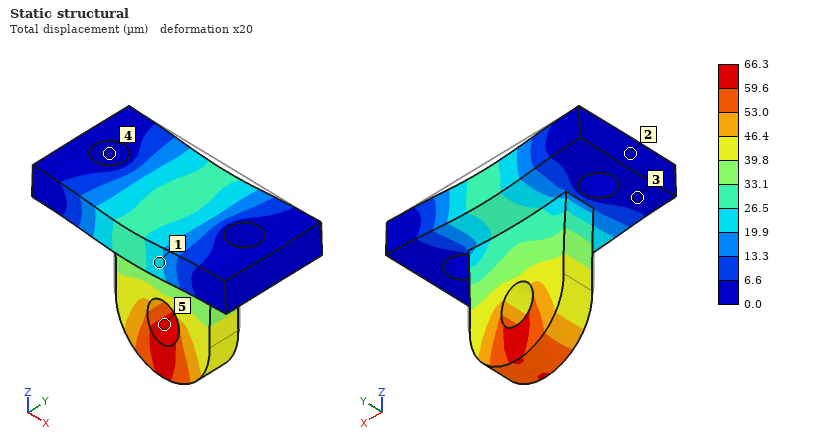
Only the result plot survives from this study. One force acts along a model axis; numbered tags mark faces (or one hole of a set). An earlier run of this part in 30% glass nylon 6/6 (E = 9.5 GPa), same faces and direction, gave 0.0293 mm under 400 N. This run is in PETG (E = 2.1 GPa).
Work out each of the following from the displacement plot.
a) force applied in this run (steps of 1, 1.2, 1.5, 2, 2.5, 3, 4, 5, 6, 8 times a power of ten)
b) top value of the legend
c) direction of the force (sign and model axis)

200 N
66.3 µm
-Z
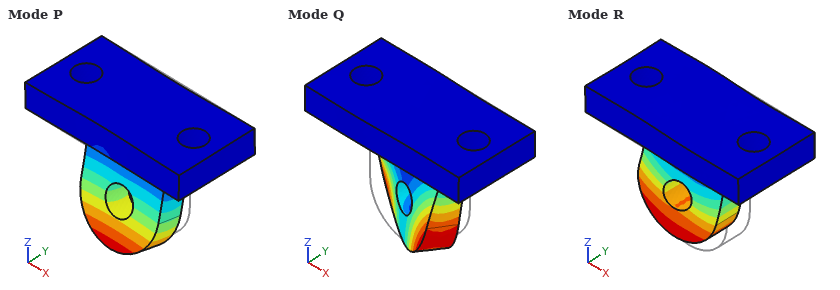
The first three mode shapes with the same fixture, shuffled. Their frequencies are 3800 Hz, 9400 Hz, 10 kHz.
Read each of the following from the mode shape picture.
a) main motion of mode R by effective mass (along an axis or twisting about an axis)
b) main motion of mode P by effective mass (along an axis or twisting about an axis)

along X
along Y
